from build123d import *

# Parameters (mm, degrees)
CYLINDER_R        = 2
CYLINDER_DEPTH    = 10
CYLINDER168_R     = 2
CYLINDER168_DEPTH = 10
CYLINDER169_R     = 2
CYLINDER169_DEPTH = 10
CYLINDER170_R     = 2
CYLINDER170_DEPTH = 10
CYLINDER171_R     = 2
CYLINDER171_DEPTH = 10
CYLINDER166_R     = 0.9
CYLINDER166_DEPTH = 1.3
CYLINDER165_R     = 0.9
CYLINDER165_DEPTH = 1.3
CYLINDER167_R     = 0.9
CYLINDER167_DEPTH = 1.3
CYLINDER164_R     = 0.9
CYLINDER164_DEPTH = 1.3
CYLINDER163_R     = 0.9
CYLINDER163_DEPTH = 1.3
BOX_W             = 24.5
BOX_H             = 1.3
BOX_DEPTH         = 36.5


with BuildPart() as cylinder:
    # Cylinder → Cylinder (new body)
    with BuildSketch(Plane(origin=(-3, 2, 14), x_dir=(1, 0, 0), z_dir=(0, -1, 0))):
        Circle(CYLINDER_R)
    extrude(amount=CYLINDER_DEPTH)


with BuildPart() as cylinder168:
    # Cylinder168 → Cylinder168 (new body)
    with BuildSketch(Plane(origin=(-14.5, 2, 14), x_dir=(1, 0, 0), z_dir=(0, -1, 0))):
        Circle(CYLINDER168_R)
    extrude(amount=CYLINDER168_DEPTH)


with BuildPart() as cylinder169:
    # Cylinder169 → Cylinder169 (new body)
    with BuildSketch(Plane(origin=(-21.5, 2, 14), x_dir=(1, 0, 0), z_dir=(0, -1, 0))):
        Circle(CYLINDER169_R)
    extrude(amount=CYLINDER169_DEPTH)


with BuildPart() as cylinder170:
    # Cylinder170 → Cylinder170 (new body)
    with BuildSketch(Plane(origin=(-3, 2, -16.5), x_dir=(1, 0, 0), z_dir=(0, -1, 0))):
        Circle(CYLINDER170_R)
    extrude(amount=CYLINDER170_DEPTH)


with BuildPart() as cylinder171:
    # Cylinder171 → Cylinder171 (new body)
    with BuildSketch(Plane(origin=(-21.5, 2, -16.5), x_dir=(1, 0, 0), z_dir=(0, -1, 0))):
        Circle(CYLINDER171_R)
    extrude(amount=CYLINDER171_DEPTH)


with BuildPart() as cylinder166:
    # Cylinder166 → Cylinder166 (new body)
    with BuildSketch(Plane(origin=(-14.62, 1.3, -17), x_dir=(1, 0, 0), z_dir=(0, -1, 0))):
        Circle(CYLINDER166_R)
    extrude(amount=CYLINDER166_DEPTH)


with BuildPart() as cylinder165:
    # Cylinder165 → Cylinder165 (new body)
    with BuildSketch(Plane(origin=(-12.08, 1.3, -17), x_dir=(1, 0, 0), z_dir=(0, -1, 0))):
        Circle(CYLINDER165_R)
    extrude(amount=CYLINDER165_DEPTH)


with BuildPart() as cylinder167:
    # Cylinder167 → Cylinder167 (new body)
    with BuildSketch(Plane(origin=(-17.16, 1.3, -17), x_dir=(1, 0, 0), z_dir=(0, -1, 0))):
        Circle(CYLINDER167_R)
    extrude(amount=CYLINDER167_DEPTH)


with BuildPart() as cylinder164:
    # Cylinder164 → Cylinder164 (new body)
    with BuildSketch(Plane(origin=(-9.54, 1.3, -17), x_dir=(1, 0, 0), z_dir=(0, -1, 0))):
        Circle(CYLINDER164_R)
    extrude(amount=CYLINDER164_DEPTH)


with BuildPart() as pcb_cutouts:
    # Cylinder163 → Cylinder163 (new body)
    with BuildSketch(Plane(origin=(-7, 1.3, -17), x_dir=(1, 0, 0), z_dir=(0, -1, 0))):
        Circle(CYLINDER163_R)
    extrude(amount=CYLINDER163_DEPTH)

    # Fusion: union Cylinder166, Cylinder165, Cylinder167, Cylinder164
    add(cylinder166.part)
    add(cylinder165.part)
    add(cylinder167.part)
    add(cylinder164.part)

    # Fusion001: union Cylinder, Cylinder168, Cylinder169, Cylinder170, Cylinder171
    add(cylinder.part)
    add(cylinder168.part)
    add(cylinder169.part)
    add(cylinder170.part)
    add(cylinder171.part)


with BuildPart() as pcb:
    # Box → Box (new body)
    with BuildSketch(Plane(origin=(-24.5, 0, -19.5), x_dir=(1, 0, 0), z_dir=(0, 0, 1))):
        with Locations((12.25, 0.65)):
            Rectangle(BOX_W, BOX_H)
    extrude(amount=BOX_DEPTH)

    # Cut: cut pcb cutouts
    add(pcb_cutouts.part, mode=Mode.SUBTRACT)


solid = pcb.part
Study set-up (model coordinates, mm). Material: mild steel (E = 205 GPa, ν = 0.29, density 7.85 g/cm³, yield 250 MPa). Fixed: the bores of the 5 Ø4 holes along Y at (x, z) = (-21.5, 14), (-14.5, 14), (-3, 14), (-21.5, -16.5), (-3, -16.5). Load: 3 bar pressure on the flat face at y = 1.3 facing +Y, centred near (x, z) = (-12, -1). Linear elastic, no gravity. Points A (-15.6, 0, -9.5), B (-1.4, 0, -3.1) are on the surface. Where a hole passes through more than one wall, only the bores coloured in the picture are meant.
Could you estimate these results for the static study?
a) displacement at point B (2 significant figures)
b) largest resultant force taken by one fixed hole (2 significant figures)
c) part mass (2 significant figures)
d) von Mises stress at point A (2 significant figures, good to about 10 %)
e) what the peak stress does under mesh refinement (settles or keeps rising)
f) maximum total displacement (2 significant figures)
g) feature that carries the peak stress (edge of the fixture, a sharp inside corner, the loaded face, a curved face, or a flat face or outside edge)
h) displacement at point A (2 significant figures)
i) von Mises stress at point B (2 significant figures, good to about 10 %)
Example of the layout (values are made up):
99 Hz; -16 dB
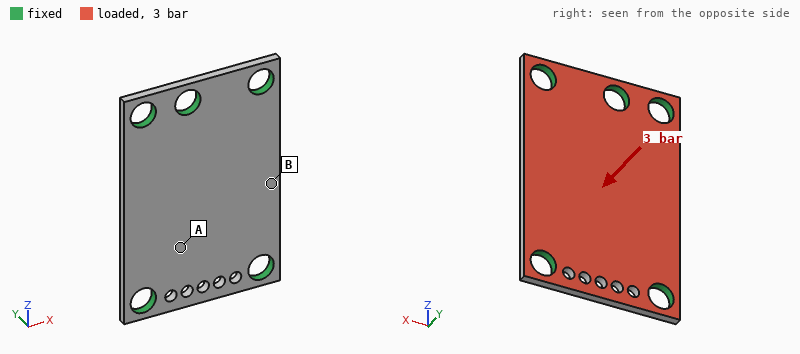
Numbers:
13 µm; 60 N; 8.4 g; 12 MPa; keeps rising; 14 µm; edge of the fixture; 8.0 µm; 36 MPa
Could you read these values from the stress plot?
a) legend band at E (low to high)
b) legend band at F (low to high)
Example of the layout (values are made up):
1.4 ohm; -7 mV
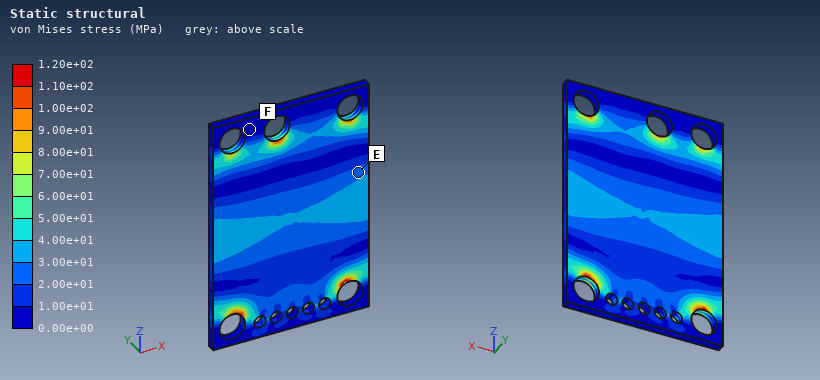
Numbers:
2.00e+01 to 3.00e+01 MPa; 0.00e+00 to 1.00e+01 MPa
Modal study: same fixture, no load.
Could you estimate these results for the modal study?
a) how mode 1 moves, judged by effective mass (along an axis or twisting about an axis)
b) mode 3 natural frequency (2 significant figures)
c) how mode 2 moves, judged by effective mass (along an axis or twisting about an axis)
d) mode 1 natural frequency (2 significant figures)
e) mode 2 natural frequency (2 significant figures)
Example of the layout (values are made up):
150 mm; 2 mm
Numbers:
along Y; 18 kHz; twisting about Z; 8500 Hz; 11 kHz
